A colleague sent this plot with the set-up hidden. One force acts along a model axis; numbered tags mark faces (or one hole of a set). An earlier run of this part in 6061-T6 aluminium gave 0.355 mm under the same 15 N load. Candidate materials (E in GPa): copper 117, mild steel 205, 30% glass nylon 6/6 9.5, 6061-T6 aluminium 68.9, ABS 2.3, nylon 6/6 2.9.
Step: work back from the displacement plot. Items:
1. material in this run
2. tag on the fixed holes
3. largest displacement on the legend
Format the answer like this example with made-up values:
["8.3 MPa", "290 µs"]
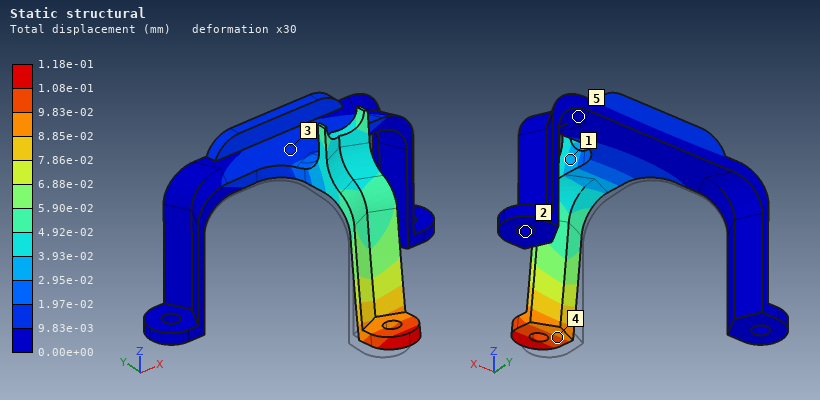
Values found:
["mild steel", "2", "1.18e-01 mm"]
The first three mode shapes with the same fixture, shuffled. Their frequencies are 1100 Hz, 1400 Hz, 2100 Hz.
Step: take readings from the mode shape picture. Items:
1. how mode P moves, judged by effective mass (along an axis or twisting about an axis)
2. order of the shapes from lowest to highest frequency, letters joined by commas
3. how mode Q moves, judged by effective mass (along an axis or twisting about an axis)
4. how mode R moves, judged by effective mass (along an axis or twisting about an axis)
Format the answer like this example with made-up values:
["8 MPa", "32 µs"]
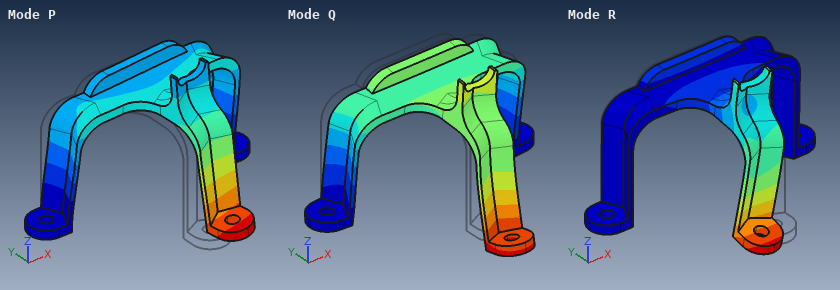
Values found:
["along X", "R, P, Q", "along Y", "along Z"]
